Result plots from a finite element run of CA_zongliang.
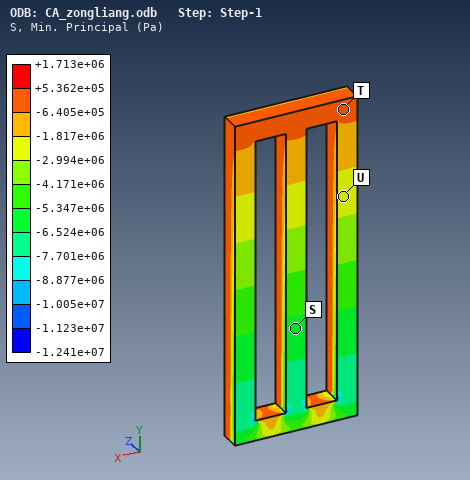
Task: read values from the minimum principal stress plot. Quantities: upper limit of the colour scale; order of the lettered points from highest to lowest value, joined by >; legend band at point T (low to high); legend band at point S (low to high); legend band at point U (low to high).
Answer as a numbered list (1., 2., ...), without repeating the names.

1. +1.713e+06 Pa
2. T > U > S
3. -6.405e+05 to +5.362e+05 Pa
4. -6.524e+06 to -5.347e+06 Pa
5. -2.994e+06 to -1.817e+06 Pa
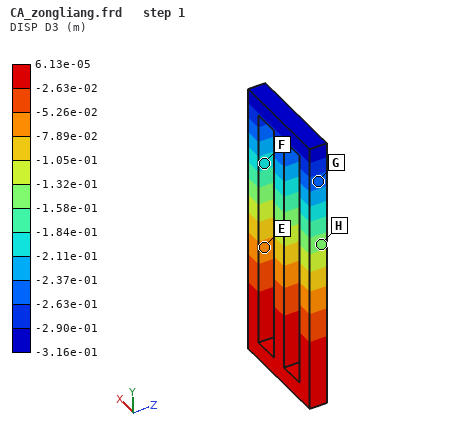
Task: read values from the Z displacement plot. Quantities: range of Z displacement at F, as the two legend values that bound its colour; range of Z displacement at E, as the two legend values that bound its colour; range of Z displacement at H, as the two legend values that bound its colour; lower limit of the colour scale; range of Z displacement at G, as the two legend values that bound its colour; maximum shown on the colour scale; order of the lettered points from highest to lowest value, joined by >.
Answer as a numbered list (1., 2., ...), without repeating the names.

1. -2.11e-01 to -1.84e-01 m
2. -7.89e-02 to -5.26e-02 m
3. -1.58e-01 to -1.32e-01 m
4. -3.16e-01 m
5. -2.63e-01 to -2.37e-01 m
6. 6.13e-05 m
7. E > H > F > G
